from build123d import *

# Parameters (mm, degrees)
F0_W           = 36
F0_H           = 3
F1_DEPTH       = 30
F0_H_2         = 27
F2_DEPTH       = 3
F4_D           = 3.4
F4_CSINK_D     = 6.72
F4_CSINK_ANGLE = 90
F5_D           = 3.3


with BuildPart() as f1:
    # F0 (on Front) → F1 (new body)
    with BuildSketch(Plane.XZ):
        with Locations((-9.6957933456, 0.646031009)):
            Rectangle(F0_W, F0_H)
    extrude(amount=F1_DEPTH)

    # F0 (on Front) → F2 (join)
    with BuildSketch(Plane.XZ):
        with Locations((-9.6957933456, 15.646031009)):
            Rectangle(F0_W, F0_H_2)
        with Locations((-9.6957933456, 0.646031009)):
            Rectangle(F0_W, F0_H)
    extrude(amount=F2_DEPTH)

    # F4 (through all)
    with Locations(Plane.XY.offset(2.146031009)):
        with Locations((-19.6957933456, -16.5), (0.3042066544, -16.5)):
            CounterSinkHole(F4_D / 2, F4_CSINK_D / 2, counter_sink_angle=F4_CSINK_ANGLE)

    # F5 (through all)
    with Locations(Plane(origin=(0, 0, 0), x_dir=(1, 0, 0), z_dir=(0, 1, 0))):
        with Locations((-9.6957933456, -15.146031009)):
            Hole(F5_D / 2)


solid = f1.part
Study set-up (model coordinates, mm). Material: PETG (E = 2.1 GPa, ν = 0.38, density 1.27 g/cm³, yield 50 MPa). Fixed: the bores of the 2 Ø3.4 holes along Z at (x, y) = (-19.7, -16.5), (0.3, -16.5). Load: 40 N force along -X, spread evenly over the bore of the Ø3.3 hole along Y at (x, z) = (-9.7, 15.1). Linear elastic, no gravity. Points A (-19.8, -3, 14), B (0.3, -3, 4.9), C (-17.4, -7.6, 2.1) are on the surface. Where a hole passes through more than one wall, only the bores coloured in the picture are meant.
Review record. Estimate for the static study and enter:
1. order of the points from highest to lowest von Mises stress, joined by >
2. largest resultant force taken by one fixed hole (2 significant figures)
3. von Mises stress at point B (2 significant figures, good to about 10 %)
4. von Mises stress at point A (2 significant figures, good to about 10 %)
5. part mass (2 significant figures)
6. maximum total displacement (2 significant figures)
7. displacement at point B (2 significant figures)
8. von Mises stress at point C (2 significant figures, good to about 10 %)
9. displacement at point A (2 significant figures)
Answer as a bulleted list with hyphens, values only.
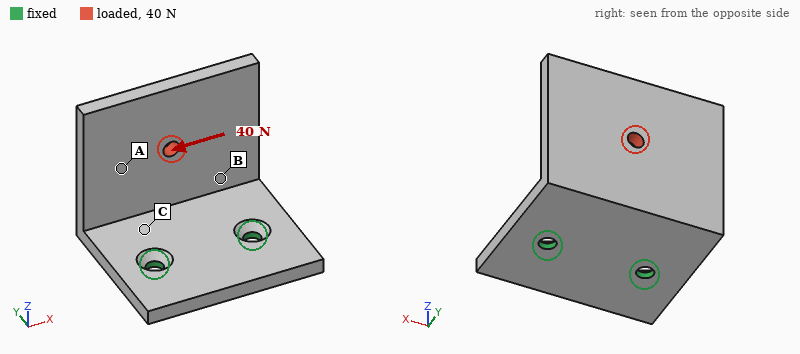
- C > B > A
- 45 N
- 3.8 MPa
- 1.6 MPa
- 7.7 g
- 0.58 mm
- 0.17 mm
- 5.6 MPa
- 0.29 mm
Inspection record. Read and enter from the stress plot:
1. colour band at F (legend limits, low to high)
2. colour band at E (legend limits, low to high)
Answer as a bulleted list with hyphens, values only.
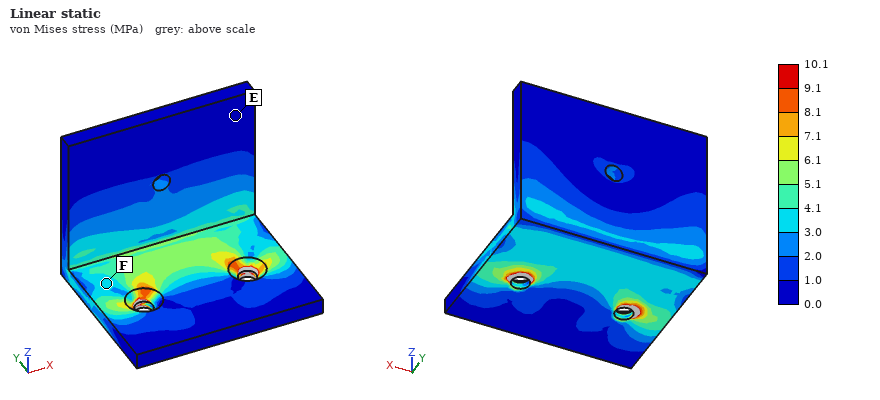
- 3.0 to 4.1 MPa
- 0.0 to 1.0 MPa
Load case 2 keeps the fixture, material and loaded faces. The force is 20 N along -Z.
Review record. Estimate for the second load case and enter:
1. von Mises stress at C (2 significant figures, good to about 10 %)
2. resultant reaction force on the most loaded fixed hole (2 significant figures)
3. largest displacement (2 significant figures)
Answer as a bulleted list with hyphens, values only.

- 1.9 MPa
- 10 N
- 0.63 mm
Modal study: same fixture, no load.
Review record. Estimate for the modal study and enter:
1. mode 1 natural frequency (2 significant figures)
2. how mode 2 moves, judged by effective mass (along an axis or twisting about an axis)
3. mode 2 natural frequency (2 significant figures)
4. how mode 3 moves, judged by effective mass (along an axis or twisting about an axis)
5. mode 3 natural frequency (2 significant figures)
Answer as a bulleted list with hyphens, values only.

- 370 Hz
- along X
- 740 Hz
- along Z
- 1200 Hz
